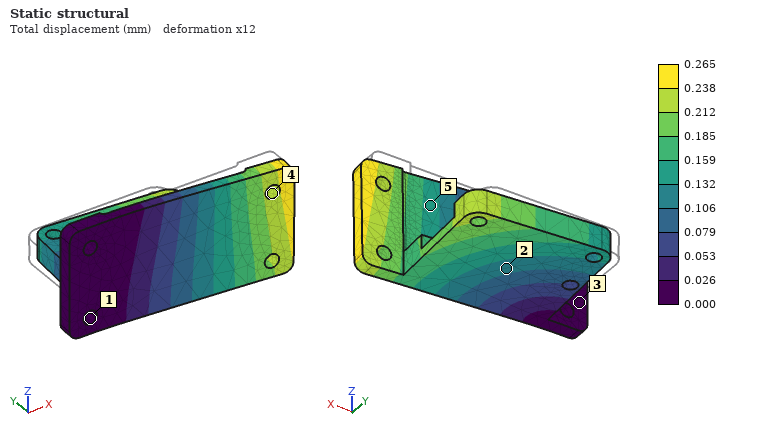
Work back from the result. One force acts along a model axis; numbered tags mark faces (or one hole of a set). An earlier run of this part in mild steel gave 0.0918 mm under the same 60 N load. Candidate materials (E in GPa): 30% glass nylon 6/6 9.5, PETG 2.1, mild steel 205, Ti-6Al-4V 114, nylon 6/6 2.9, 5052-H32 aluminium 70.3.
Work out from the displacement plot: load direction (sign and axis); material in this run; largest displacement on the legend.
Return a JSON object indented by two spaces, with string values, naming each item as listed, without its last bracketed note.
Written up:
{
  "load direction": "-Y",
  "material in this run": "5052-H32 aluminium",
  "largest displacement on the legend": "0.265 mm"
}
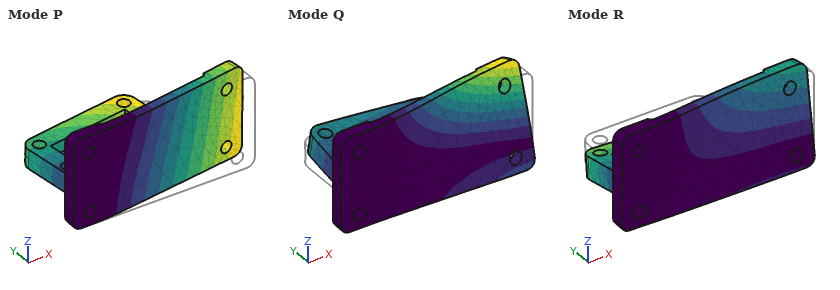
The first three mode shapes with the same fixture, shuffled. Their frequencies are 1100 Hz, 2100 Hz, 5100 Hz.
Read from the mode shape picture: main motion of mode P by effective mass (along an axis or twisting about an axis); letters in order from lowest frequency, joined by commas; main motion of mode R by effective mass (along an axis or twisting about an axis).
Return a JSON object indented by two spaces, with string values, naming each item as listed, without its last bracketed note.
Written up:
{
  "main motion of mode P by effective mass": "along Y",
  "letters in order from lowest frequency, joined by commas": "P, R, Q",
  "main motion of mode R by effective mass": "along Z"
}
